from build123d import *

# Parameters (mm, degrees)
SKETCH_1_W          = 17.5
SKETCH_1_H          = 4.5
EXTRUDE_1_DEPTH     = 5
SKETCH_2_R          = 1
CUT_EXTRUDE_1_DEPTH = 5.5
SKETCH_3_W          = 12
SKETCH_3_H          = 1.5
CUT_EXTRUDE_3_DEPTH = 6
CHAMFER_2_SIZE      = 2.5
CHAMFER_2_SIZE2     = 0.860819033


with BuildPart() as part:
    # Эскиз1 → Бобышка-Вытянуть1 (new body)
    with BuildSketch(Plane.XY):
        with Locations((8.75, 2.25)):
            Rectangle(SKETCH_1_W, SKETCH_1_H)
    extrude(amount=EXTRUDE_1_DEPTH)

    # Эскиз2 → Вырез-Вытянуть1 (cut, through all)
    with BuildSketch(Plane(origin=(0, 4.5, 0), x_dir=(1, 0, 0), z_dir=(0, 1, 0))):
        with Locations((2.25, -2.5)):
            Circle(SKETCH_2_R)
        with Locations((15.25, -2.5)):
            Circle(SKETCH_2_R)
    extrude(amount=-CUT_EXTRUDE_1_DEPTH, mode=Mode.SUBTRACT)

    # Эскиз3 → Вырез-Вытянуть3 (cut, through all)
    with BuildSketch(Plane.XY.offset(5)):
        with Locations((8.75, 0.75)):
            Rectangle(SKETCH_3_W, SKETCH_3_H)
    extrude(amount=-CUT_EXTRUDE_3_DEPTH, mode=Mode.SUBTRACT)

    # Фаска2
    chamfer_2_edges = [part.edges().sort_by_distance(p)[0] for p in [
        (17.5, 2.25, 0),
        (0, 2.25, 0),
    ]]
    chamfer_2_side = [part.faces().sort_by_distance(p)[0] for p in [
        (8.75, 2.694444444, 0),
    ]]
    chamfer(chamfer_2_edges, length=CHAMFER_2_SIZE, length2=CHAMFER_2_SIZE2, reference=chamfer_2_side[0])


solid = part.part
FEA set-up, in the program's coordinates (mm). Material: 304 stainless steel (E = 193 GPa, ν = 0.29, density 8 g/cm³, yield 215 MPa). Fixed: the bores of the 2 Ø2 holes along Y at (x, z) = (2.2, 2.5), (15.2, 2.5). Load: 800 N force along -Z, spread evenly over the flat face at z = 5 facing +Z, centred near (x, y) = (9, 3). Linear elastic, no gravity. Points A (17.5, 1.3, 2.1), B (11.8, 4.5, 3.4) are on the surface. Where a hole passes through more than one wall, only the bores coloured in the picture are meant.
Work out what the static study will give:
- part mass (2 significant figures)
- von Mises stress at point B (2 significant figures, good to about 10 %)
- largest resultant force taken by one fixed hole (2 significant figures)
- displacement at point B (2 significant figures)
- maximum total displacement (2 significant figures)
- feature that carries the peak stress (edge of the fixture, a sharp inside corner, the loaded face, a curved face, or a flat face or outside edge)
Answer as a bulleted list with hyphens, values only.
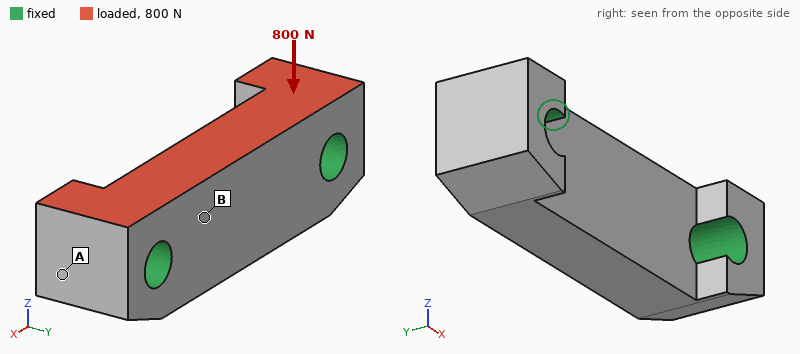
- 2.1 g
- 21 MPa
- 400 N
- 0.91 µm
- 1.4 µm
- edge of the fixture
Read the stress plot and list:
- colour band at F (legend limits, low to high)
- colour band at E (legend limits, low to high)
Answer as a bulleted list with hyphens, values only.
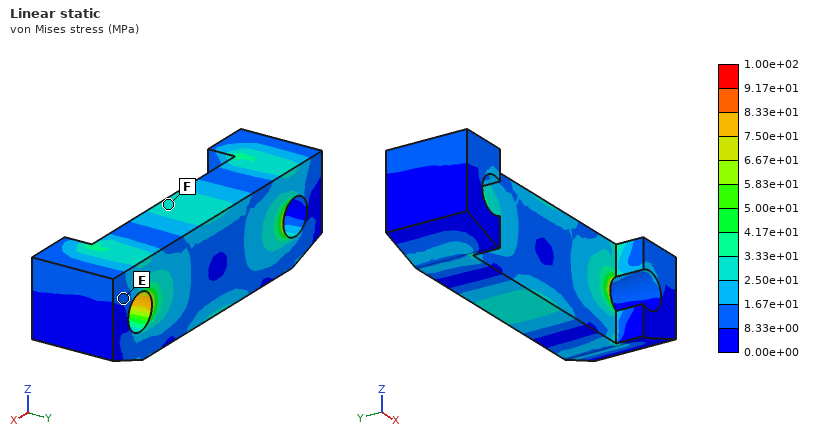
- 2.50e+01 to 3.33e+01 MPa
- 8.33e+00 to 1.67e+01 MPa
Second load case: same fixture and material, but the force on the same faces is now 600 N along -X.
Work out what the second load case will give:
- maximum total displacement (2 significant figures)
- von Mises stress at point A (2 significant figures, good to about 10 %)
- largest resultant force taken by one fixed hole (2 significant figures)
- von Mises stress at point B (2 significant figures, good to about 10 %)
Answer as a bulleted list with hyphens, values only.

- 0.67 µm
- 11 MPa
- 310 N
- 15 MPa
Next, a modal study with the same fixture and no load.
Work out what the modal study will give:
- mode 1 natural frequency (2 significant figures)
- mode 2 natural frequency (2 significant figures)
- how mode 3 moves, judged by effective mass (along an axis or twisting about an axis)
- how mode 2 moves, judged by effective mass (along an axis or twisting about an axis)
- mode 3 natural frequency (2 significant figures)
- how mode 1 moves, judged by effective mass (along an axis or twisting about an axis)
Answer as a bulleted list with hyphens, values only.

- 78 kHz
- 87 kHz
- twisting about X
- along Z
- 110 kHz
- along Y
